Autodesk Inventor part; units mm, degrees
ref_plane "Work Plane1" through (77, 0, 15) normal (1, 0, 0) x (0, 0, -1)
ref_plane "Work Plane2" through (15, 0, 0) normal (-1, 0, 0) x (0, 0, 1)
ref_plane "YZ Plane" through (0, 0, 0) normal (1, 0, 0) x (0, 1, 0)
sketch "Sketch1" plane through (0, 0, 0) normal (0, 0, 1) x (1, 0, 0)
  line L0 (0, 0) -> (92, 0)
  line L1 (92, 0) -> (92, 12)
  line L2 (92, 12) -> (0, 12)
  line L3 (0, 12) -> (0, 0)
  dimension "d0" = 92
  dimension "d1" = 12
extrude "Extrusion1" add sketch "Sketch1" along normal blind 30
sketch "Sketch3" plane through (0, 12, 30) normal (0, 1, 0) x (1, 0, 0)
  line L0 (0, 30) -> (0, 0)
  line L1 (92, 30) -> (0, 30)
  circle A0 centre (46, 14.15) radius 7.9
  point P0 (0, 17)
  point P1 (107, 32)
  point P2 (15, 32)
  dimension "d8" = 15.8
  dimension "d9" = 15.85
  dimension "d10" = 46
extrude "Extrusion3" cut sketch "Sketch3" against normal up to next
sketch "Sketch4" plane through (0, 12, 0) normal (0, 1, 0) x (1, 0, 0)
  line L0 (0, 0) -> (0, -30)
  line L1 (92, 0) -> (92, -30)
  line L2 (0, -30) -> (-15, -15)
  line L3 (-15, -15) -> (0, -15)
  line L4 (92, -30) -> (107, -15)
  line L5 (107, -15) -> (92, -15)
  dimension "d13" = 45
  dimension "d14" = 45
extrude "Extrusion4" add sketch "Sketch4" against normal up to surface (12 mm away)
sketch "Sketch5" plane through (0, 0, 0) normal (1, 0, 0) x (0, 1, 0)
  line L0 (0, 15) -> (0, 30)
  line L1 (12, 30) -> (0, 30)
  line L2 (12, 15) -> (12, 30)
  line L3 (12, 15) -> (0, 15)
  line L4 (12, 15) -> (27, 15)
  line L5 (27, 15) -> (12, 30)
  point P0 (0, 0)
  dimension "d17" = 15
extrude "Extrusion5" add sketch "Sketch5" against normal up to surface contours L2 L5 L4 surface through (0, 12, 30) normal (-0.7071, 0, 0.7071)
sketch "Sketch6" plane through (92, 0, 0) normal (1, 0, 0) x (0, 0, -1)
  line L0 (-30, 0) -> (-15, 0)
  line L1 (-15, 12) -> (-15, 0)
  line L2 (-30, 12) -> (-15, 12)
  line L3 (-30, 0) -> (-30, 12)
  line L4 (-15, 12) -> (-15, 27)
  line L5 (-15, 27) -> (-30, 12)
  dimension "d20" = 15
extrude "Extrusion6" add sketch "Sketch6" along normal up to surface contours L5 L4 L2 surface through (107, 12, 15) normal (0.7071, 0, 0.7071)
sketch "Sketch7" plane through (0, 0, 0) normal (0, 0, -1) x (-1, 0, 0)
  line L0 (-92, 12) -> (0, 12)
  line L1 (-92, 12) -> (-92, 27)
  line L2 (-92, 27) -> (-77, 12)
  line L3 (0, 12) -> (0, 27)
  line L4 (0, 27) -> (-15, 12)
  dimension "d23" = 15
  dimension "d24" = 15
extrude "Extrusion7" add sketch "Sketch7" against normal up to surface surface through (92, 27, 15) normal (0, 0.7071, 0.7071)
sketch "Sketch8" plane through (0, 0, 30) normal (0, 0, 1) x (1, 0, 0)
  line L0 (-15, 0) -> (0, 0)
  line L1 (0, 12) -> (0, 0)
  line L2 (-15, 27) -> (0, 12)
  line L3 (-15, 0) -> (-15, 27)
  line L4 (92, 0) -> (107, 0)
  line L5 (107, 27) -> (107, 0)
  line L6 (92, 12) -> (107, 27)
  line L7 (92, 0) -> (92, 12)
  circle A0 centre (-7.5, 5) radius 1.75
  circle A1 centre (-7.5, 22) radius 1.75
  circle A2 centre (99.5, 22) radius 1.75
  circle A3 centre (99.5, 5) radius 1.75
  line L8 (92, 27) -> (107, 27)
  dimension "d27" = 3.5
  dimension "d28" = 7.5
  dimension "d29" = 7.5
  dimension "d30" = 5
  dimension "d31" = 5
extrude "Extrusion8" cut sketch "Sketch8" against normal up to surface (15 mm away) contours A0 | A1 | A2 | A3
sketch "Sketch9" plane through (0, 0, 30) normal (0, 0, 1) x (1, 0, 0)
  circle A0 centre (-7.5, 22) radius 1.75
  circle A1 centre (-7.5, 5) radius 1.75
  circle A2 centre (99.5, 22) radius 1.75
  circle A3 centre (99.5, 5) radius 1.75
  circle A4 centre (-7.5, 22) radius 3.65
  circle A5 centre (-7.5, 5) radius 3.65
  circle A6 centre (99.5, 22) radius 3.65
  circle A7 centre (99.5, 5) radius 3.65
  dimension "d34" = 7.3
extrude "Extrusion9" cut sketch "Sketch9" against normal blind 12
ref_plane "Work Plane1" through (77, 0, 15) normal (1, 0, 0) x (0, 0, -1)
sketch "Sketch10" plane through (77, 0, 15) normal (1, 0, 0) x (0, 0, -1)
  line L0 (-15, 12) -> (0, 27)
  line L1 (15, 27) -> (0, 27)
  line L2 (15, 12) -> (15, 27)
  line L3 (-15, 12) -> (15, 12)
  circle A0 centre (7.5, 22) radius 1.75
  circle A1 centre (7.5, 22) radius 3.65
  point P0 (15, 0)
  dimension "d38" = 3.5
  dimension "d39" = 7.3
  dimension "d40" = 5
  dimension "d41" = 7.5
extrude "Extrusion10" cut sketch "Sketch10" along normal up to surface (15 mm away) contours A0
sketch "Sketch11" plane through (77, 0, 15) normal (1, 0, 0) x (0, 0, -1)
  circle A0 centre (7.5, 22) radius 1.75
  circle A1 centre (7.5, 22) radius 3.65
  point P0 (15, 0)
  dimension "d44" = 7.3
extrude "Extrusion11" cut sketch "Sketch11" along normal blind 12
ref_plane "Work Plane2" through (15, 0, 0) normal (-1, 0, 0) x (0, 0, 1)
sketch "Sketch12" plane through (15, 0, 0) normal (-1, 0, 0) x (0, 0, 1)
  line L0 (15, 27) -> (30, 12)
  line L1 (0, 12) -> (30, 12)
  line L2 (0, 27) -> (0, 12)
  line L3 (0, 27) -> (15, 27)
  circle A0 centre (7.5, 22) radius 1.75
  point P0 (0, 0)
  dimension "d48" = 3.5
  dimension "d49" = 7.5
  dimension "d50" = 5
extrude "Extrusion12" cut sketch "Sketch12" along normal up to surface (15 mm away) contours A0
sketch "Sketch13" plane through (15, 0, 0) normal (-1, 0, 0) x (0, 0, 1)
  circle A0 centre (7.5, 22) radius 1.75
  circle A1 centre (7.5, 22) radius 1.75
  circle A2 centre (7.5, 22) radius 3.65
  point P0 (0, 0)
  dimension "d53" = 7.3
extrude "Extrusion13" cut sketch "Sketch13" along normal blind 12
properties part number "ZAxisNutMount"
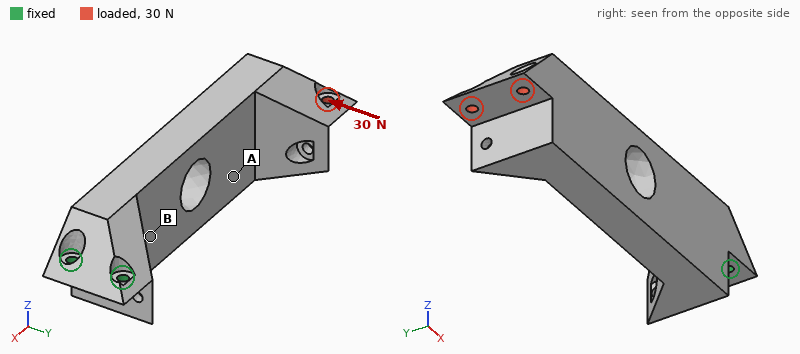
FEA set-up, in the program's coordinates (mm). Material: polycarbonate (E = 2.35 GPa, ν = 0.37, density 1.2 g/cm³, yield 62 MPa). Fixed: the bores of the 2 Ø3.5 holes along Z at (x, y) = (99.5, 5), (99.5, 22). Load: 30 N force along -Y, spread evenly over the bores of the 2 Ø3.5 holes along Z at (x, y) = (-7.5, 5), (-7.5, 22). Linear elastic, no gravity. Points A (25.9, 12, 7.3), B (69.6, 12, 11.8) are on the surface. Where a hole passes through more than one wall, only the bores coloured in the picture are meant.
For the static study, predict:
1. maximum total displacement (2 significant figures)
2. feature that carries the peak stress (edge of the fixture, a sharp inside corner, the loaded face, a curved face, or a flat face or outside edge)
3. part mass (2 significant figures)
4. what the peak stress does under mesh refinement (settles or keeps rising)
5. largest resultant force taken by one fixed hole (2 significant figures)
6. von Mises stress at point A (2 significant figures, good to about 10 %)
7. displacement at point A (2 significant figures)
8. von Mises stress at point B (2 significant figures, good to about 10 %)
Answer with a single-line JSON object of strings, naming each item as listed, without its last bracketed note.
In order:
{"maximum total displacement": "1.5 mm", "feature that carries the peak stress": "edge of the fixture", "part mass": "49 g", "what the peak stress does under mesh refinement": "keeps rising", "largest resultant force taken by one fixed hole": "180 N", "von Mises stress at point A": "1.5 MPa", "displacement at point A": "0.67 mm", "von Mises stress at point B": "3.1 MPa"}
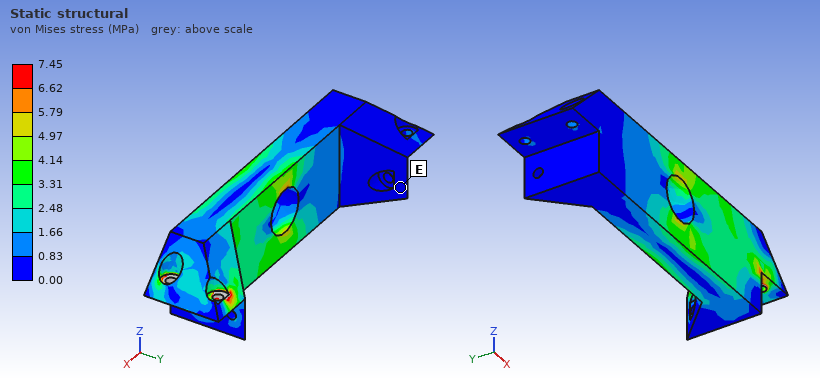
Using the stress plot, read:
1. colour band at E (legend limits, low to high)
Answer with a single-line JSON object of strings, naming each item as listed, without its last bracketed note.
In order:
{"colour band at E": "0.00 to 0.83 MPa"}
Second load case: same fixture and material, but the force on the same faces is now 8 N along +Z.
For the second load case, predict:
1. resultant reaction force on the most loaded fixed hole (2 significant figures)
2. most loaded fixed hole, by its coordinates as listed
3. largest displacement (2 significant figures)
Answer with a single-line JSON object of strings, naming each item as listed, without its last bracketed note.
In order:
{"resultant reaction force on the most loaded fixed hole": "7.4 N", "most loaded fixed hole, by its coordinates as listed": "(99.5, 5)", "largest displacement": "1.3 mm"}
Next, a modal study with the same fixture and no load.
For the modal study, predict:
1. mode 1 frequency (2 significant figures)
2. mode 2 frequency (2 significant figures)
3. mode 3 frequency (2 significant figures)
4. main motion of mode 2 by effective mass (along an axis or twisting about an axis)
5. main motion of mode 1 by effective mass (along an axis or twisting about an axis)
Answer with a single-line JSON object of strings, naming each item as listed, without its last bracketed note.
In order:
{"mode 1 frequency": "99 Hz", "mode 2 frequency": "220 Hz", "mode 3 frequency": "960 Hz", "main motion of mode 2 by effective mass": "along Y", "main motion of mode 1 by effective mass": "along Z"}
